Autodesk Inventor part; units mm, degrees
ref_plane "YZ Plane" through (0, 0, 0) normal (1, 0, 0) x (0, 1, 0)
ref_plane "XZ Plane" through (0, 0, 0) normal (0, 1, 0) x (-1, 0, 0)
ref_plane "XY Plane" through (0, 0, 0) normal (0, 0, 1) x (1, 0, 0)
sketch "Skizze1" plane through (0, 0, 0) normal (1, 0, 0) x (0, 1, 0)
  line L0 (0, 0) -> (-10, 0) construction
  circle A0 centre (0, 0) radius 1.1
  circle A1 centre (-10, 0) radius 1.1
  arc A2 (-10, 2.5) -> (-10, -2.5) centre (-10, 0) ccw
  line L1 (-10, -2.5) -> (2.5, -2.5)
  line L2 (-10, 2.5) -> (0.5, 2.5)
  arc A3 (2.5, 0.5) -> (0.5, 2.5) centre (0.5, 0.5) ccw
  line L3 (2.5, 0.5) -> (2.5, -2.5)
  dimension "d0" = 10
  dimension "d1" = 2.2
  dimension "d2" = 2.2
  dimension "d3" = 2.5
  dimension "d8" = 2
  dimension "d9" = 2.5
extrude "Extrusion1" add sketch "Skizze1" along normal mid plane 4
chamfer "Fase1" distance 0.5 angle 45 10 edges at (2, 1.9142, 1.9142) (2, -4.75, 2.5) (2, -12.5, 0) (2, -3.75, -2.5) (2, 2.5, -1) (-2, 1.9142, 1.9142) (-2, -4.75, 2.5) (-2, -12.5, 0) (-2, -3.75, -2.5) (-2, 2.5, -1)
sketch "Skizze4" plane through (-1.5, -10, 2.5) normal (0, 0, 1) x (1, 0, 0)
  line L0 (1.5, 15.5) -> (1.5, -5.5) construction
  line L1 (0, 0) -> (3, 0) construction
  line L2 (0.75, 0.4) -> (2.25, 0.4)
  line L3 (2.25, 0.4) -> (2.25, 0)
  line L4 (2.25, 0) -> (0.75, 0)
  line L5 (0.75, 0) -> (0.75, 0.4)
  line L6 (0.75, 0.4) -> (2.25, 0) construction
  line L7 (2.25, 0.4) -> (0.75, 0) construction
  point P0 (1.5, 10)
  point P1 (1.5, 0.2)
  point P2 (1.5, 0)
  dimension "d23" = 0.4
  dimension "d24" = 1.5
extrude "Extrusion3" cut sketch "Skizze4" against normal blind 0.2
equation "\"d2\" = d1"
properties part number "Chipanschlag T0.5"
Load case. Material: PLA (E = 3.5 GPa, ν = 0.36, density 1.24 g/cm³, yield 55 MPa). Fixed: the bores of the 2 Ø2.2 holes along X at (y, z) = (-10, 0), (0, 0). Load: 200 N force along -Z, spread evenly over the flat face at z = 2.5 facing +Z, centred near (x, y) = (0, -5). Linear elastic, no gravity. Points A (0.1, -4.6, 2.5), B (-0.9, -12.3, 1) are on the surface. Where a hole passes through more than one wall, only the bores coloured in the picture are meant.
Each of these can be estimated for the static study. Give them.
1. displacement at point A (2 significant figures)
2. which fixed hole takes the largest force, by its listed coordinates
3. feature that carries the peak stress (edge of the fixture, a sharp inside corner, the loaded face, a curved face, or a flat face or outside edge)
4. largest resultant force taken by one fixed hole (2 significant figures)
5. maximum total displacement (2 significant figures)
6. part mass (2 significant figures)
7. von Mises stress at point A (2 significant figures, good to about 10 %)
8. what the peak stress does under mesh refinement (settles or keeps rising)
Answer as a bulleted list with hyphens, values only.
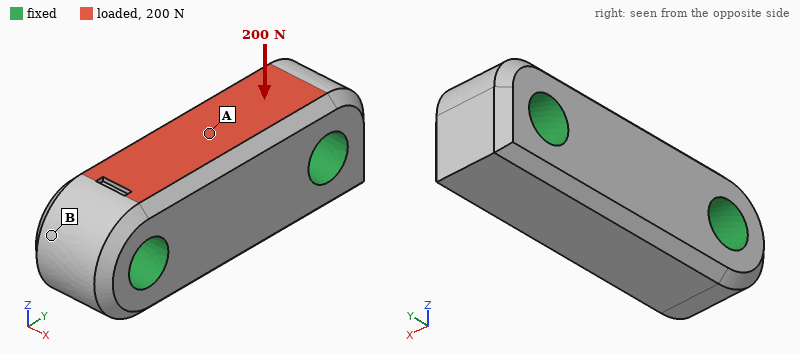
- 14 µm
- (0, 0)
- edge of the fixture
- 110 N
- 14 µm
- 0.31 g
- 6.6 MPa
- keeps rising
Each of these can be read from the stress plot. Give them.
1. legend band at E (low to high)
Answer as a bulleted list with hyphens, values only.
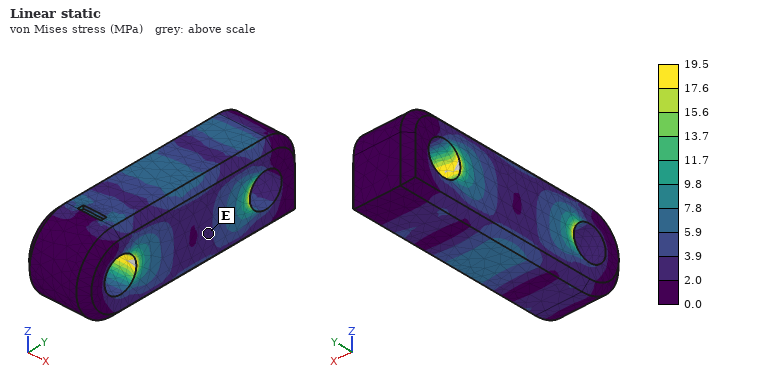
- 2.0 to 3.9 MPa
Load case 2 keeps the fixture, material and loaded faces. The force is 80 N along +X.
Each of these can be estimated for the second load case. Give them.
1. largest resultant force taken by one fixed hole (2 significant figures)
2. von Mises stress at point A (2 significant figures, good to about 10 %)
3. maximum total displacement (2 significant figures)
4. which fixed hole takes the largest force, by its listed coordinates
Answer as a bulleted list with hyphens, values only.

- 43 N
- 4.6 MPa
- 15 µm
- (0, 0)
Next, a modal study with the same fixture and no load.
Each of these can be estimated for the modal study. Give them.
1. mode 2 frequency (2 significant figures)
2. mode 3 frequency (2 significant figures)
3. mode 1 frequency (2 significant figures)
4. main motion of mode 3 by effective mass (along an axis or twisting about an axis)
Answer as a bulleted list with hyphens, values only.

- 46 kHz
- 53 kHz
- 45 kHz
- twisting about Y
